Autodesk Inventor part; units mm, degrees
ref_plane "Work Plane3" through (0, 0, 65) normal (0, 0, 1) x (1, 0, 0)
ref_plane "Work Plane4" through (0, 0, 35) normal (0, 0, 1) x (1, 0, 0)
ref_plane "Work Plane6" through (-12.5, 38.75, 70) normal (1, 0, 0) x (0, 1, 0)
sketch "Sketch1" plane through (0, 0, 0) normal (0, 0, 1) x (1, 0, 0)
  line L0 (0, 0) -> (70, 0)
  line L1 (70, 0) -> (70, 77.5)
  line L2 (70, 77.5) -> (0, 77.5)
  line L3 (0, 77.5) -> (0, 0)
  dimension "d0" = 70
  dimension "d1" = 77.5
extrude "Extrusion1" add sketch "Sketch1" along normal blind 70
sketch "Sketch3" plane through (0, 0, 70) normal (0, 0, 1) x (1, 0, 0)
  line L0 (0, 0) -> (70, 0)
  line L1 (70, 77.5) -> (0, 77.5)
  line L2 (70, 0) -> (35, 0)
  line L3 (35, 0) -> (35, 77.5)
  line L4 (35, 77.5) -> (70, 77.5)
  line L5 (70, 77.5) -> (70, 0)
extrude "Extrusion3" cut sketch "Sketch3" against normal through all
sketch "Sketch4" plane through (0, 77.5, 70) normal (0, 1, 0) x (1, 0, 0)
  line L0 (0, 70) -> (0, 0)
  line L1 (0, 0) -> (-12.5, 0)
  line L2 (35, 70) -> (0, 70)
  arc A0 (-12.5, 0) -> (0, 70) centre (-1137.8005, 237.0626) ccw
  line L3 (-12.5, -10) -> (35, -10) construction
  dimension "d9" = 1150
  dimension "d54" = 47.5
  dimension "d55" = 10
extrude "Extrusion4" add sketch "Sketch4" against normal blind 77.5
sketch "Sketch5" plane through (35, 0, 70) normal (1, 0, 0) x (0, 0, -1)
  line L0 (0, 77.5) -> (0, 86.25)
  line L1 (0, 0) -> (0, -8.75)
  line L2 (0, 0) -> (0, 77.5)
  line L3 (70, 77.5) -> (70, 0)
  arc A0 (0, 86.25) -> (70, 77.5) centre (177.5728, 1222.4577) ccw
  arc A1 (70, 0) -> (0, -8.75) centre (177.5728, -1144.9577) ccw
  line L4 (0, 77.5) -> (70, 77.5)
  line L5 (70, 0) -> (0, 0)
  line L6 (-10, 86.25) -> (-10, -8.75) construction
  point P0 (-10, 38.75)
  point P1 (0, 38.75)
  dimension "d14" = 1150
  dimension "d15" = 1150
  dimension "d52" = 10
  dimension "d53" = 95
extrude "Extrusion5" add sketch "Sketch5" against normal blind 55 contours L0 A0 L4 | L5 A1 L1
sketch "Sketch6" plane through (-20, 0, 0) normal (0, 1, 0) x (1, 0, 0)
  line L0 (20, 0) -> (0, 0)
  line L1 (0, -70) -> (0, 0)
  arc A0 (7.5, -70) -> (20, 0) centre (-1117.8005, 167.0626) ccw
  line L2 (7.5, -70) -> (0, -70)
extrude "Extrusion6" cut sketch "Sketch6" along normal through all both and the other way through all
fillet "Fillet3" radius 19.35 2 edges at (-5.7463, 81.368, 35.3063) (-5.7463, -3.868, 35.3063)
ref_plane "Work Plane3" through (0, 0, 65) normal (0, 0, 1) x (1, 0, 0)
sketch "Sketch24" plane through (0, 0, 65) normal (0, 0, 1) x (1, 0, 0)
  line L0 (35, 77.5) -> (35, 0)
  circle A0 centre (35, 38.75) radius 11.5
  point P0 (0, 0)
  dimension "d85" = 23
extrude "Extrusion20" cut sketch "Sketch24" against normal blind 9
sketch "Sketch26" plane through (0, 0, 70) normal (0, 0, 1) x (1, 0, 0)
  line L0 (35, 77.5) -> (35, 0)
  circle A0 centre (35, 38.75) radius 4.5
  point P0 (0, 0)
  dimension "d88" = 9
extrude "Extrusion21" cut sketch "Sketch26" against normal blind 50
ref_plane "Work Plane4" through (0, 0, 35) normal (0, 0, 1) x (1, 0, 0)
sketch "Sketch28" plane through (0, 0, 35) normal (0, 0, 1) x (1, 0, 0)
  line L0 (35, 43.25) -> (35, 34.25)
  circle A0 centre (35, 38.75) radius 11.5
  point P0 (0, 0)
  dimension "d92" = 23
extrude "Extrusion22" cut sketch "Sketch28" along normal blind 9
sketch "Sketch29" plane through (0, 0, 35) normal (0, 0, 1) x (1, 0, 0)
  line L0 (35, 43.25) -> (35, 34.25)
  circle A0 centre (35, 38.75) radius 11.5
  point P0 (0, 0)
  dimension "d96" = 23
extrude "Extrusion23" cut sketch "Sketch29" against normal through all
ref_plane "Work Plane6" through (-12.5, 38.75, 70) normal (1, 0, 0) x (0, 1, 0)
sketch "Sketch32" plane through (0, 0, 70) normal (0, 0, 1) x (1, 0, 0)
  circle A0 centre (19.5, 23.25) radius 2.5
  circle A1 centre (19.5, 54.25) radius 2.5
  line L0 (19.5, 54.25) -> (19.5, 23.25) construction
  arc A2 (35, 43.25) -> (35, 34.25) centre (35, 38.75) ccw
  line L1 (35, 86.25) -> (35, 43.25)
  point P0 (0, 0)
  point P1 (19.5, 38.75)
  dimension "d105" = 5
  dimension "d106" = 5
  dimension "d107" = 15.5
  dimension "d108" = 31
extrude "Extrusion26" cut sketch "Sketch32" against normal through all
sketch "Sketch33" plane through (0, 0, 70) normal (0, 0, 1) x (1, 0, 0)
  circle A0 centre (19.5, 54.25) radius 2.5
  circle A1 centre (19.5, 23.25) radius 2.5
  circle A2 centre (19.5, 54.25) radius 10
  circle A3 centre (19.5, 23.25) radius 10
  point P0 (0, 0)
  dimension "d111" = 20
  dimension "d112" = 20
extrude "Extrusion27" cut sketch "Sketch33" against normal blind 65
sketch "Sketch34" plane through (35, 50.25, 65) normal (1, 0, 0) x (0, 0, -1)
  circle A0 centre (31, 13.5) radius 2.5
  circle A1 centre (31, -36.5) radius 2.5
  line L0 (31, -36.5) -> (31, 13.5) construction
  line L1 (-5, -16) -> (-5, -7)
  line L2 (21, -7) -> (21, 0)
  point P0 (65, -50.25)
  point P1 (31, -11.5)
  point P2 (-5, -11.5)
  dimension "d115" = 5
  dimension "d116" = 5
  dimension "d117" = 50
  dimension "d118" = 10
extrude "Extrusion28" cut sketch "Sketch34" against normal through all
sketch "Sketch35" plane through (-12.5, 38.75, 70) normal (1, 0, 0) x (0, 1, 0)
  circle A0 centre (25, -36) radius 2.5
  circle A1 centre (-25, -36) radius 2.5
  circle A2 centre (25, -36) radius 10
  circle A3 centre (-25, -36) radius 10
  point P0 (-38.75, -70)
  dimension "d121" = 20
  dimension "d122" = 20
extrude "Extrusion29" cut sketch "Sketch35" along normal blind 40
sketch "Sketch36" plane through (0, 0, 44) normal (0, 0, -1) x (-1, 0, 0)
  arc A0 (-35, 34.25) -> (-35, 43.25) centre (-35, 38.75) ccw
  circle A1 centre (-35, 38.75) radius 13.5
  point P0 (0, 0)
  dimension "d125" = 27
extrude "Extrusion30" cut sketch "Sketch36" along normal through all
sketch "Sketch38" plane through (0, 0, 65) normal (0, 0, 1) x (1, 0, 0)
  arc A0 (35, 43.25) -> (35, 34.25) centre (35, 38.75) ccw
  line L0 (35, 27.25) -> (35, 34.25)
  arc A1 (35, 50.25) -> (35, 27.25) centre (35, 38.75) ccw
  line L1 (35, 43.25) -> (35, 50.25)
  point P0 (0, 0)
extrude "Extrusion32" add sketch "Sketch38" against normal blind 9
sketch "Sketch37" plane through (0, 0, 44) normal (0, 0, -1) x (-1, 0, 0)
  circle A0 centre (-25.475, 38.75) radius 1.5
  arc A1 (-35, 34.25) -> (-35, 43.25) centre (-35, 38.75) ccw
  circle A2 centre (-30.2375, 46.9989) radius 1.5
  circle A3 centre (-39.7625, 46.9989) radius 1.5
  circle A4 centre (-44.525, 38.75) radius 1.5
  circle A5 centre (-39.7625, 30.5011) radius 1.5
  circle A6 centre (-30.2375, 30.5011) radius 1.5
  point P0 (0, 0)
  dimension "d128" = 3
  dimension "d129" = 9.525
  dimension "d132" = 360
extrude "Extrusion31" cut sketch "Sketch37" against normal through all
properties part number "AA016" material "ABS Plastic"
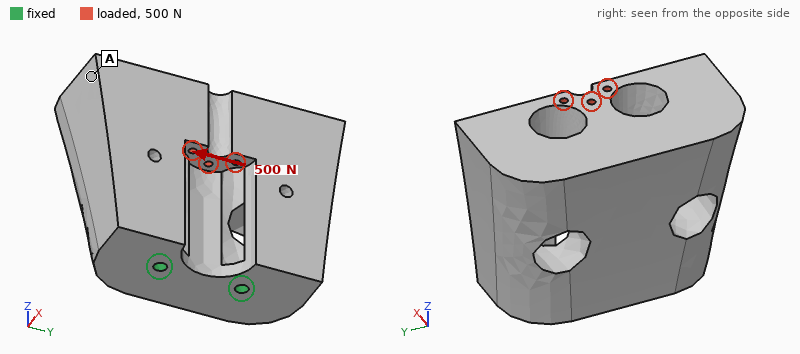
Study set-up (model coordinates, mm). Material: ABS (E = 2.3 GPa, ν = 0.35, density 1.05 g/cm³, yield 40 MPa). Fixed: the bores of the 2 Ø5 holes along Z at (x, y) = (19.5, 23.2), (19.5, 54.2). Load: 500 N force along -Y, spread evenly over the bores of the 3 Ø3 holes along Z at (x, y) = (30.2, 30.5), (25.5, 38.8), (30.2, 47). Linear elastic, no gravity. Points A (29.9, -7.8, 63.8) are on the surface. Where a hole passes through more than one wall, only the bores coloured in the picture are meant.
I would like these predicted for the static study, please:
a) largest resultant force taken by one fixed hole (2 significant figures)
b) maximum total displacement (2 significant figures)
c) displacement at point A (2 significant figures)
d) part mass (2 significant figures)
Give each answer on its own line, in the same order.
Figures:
800 N
0.98 mm
0.90 mm
170 g
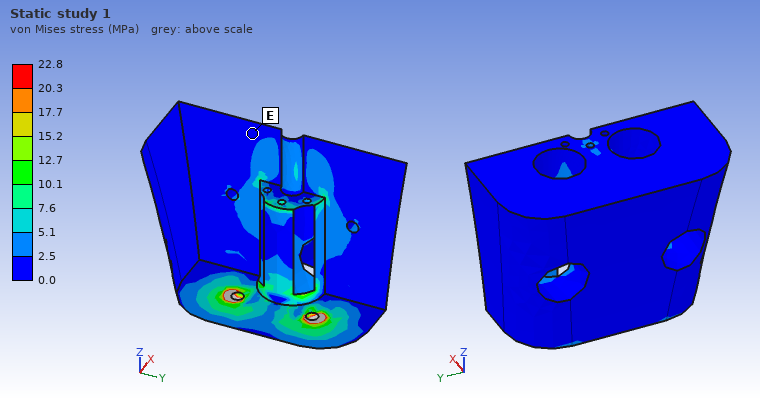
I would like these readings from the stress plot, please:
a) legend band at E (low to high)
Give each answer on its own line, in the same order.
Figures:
0.0 to 2.5 MPa
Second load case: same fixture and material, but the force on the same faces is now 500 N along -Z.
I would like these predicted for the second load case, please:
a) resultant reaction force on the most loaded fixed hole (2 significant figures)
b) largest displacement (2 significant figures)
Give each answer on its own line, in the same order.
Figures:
250 N
0.84 mm
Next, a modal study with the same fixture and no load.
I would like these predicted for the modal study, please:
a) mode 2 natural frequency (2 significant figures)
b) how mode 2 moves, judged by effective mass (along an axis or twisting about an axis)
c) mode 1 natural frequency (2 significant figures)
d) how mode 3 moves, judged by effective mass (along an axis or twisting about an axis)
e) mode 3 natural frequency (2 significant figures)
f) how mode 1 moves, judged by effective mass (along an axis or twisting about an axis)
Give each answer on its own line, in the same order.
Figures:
410 Hz
along Y
170 Hz
twisting about Z
800 Hz
along X
